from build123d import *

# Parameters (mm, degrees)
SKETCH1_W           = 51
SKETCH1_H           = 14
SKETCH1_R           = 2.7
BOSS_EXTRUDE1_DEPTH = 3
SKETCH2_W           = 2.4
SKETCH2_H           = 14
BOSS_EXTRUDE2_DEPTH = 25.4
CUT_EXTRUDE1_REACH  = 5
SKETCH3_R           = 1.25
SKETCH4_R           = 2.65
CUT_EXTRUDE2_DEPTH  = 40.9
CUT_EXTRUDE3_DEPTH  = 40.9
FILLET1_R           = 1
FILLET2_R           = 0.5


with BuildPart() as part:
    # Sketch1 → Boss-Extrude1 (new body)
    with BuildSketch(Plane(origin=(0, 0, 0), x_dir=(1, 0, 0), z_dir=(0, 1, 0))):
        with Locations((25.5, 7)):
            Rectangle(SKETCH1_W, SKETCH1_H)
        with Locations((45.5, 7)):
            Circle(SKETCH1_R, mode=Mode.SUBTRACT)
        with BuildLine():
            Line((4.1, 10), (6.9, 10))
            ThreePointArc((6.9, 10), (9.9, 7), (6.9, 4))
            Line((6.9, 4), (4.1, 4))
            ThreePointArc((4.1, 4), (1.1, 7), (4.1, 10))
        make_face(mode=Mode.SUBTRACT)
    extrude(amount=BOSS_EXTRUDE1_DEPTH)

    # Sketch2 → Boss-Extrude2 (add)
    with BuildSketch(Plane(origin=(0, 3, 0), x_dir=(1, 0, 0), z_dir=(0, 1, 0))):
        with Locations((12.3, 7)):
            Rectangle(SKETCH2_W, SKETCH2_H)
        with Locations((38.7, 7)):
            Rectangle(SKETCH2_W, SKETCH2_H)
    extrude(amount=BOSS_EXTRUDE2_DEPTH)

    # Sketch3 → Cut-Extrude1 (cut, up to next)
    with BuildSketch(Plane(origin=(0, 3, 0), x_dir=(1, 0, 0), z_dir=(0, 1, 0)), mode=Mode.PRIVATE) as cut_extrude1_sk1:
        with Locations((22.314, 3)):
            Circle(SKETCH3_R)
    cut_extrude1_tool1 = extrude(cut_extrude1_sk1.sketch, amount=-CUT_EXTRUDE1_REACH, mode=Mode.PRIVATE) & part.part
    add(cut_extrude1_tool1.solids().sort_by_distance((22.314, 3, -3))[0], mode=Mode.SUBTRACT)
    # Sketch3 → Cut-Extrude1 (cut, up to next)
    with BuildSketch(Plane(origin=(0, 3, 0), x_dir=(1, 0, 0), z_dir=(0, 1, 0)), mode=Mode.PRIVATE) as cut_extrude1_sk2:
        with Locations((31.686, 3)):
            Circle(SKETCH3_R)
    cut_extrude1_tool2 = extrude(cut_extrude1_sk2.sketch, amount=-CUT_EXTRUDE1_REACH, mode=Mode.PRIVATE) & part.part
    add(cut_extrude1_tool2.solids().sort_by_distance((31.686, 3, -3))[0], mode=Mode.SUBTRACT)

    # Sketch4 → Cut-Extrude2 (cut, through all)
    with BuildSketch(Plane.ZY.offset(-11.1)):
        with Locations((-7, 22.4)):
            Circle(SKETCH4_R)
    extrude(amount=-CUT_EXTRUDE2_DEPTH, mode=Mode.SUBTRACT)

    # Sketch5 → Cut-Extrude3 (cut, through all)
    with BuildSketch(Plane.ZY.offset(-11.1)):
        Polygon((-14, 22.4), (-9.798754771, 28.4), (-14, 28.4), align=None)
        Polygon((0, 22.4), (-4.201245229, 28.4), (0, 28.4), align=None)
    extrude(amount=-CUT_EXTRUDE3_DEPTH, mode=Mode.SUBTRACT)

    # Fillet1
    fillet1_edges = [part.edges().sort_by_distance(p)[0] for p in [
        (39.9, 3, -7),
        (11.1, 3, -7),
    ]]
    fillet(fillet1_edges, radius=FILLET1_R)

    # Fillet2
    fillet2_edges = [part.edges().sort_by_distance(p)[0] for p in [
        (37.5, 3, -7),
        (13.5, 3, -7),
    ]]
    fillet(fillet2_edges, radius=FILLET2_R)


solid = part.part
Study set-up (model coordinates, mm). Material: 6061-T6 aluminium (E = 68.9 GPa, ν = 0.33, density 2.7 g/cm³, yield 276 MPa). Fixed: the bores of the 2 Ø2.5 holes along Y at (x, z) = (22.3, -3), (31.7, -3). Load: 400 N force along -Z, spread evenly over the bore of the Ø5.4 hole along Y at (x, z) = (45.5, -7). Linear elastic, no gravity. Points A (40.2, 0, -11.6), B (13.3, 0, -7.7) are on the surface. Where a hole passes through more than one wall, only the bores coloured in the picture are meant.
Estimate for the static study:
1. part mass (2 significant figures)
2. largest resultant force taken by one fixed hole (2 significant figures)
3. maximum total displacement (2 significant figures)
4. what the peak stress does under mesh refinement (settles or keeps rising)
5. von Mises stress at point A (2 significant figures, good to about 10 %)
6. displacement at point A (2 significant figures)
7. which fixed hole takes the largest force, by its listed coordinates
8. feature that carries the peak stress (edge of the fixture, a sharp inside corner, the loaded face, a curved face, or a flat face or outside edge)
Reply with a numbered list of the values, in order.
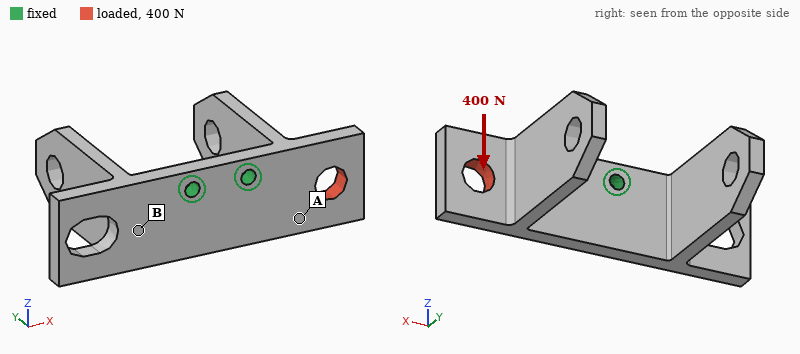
1. 9.2 g
2. 840 N
3. 40 µm
4. keeps rising
5. 18 MPa
6. 18 µm
7. (31.7, -3)
8. edge of the fixture
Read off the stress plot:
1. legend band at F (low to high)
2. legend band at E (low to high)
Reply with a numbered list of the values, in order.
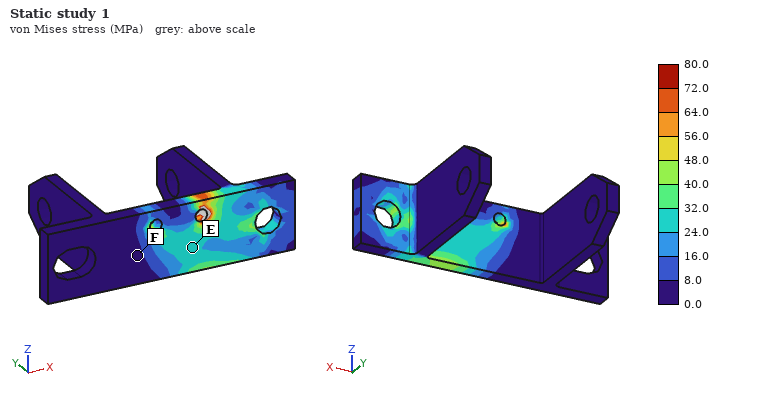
1. 0.0 to 8.0 MPa
2. 24.0 to 32.0 MPa
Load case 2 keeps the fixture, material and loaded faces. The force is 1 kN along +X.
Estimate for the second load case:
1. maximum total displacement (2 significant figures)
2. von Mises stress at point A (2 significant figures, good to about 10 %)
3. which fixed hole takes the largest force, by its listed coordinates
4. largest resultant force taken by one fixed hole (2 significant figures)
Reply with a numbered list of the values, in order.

1. 17 µm
2. 29 MPa
3. (31.7, -3)
4. 790 N
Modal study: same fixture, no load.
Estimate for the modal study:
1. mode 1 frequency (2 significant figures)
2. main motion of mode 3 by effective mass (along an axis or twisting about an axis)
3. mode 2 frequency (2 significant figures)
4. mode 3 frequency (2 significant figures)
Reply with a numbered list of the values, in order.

1. 2400 Hz
2. along Z
3. 2700 Hz
4. 3800 Hz
